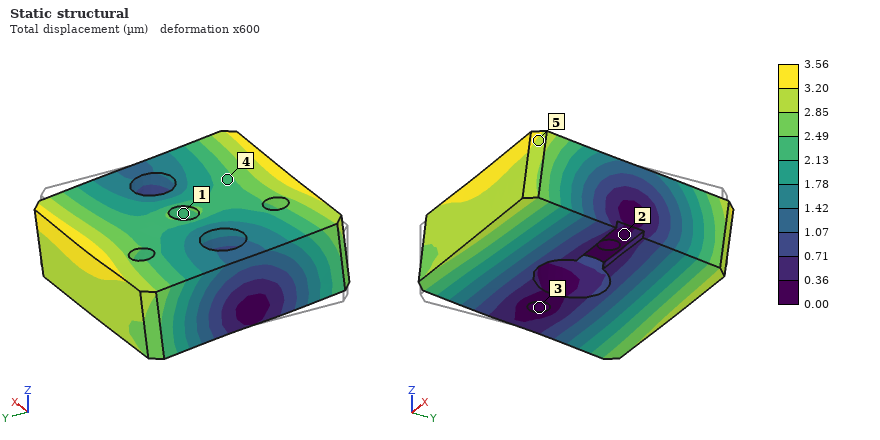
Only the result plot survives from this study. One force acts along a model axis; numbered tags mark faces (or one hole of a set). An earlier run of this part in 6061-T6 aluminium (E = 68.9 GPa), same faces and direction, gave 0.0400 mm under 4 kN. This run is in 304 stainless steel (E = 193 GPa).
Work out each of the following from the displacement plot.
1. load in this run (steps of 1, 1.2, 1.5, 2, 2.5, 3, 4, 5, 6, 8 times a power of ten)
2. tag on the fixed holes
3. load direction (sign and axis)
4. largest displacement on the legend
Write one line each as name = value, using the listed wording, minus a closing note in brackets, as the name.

load in this run = 1 kN
tag on the fixed holes = 3
load direction = +Y
largest displacement on the legend = 3.56 µm
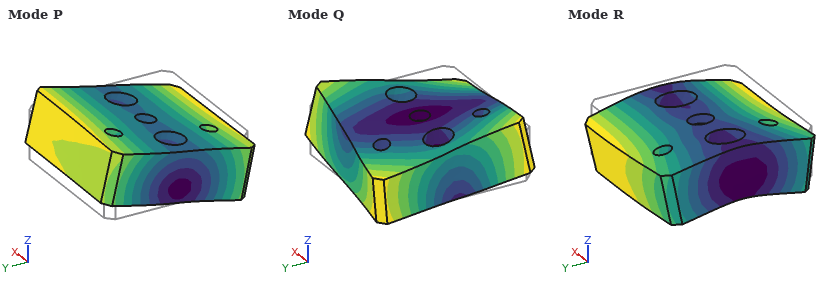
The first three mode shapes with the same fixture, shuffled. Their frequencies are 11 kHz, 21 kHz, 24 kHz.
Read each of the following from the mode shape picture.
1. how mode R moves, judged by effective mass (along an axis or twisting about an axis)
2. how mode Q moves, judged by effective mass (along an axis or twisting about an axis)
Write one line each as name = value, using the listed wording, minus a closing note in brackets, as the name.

how mode R moves, judged by effective mass = along Z
how mode Q moves, judged by effective mass = twisting about Z
